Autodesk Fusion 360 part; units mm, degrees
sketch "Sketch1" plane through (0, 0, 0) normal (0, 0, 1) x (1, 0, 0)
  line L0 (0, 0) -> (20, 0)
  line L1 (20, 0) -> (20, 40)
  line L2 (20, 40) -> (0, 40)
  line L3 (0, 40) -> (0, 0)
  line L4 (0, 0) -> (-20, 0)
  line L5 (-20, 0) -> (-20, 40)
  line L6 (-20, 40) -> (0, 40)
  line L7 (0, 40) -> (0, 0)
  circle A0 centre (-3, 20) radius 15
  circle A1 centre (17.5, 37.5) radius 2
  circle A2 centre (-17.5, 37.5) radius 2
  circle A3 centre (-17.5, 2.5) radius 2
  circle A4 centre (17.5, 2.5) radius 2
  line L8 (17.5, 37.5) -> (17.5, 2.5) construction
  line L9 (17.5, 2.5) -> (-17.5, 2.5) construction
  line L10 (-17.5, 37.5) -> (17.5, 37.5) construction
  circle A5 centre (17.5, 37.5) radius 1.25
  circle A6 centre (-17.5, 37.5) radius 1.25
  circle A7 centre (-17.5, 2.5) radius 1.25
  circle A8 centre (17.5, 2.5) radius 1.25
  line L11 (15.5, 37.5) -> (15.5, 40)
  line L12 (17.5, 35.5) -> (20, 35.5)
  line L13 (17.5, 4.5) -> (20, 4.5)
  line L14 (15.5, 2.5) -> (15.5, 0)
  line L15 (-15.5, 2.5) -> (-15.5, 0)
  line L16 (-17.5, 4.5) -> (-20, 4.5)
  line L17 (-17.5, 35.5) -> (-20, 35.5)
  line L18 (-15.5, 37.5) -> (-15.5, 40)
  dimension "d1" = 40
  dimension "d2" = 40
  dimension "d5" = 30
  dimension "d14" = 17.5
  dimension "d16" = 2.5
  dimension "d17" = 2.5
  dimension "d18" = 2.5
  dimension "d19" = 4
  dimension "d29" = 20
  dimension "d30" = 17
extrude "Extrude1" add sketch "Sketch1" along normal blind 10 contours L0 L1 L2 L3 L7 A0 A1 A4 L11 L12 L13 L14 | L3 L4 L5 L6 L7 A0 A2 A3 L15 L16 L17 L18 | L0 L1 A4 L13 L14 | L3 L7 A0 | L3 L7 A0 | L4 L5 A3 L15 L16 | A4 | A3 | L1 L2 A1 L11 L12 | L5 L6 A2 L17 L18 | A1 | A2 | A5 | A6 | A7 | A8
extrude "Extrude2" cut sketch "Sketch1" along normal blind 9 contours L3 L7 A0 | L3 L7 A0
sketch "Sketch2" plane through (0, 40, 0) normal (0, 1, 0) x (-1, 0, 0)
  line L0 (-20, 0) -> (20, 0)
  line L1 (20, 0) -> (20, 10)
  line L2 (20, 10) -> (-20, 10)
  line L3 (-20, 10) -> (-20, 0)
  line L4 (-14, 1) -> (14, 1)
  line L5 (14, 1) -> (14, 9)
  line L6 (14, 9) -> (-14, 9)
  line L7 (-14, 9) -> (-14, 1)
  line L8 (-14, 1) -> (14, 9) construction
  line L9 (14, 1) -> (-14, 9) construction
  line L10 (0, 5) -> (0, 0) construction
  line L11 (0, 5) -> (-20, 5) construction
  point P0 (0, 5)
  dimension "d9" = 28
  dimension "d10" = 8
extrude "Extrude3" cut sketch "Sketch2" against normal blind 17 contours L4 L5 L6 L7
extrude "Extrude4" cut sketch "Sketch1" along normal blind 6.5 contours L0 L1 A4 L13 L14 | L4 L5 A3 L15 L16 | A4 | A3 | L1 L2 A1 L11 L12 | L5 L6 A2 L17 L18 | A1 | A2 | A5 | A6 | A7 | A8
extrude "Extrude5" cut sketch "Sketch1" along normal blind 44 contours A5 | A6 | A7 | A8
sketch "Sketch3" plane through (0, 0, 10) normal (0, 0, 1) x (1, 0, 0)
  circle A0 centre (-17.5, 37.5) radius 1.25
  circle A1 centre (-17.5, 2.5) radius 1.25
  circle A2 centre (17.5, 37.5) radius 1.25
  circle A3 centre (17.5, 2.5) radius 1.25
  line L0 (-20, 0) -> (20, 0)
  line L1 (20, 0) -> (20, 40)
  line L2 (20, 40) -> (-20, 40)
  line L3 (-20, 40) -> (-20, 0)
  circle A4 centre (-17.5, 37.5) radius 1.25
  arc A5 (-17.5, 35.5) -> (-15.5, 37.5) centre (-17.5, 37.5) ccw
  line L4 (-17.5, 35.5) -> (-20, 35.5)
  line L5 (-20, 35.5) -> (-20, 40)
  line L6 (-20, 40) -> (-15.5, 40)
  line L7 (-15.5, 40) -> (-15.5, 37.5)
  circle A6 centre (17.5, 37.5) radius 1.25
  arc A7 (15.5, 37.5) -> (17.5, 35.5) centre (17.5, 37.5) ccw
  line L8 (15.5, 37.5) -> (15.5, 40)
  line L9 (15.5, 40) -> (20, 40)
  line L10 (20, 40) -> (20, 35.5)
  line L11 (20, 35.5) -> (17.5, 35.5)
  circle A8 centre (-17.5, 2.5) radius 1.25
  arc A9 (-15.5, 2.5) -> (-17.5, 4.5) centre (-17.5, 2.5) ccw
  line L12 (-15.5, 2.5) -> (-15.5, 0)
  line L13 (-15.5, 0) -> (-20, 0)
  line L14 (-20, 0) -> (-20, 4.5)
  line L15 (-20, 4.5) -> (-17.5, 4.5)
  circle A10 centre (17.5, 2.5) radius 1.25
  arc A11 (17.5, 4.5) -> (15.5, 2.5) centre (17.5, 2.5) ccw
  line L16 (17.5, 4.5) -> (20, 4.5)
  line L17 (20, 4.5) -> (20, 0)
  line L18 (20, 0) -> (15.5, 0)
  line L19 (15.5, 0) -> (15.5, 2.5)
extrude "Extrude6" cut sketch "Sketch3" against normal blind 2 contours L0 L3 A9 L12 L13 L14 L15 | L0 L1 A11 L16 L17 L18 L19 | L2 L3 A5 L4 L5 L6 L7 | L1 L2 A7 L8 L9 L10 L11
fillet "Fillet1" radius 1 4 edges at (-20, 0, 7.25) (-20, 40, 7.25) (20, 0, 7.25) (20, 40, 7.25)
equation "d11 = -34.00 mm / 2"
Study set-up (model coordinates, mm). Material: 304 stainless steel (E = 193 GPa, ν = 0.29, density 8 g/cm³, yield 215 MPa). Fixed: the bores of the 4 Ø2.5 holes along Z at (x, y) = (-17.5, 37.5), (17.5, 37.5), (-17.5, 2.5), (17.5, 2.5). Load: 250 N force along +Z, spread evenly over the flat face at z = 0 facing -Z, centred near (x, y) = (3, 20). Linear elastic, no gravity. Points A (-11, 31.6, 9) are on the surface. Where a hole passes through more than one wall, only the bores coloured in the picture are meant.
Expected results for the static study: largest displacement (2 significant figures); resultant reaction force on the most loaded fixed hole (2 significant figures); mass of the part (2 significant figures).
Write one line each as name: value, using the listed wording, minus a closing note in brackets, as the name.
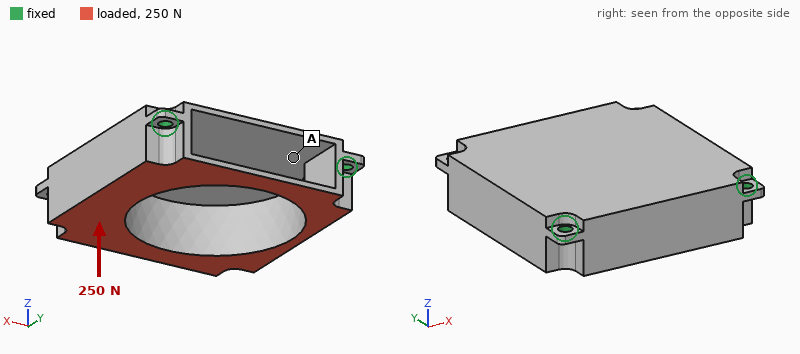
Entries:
largest displacement: 32 µm
resultant reaction force on the most loaded fixed hole: 79 N
mass of the part: 57 g
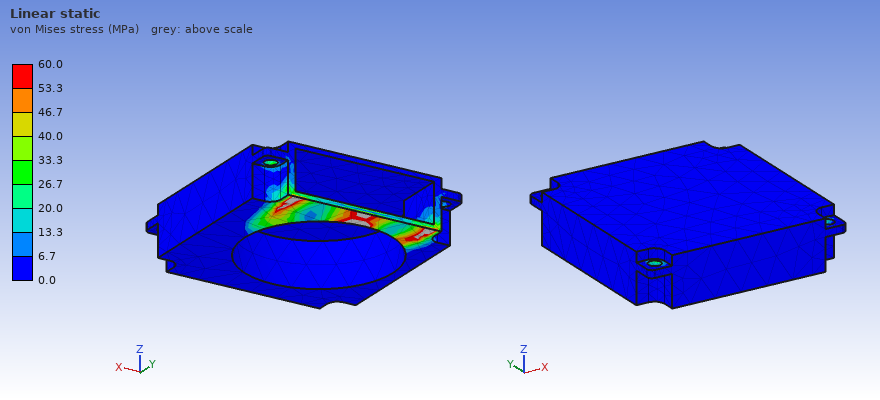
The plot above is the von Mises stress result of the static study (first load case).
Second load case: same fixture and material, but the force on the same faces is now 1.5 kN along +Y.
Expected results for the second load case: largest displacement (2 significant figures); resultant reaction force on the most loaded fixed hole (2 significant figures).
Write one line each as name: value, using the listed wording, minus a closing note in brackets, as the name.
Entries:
largest displacement: 14 µm
resultant reaction force on the most loaded fixed hole: 520 N
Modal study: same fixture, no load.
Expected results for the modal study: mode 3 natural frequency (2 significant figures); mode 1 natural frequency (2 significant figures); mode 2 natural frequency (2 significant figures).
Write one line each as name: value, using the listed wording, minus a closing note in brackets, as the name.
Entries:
mode 3 natural frequency: 9200 Hz
mode 1 natural frequency: 6300 Hz
mode 2 natural frequency: 6700 Hz
